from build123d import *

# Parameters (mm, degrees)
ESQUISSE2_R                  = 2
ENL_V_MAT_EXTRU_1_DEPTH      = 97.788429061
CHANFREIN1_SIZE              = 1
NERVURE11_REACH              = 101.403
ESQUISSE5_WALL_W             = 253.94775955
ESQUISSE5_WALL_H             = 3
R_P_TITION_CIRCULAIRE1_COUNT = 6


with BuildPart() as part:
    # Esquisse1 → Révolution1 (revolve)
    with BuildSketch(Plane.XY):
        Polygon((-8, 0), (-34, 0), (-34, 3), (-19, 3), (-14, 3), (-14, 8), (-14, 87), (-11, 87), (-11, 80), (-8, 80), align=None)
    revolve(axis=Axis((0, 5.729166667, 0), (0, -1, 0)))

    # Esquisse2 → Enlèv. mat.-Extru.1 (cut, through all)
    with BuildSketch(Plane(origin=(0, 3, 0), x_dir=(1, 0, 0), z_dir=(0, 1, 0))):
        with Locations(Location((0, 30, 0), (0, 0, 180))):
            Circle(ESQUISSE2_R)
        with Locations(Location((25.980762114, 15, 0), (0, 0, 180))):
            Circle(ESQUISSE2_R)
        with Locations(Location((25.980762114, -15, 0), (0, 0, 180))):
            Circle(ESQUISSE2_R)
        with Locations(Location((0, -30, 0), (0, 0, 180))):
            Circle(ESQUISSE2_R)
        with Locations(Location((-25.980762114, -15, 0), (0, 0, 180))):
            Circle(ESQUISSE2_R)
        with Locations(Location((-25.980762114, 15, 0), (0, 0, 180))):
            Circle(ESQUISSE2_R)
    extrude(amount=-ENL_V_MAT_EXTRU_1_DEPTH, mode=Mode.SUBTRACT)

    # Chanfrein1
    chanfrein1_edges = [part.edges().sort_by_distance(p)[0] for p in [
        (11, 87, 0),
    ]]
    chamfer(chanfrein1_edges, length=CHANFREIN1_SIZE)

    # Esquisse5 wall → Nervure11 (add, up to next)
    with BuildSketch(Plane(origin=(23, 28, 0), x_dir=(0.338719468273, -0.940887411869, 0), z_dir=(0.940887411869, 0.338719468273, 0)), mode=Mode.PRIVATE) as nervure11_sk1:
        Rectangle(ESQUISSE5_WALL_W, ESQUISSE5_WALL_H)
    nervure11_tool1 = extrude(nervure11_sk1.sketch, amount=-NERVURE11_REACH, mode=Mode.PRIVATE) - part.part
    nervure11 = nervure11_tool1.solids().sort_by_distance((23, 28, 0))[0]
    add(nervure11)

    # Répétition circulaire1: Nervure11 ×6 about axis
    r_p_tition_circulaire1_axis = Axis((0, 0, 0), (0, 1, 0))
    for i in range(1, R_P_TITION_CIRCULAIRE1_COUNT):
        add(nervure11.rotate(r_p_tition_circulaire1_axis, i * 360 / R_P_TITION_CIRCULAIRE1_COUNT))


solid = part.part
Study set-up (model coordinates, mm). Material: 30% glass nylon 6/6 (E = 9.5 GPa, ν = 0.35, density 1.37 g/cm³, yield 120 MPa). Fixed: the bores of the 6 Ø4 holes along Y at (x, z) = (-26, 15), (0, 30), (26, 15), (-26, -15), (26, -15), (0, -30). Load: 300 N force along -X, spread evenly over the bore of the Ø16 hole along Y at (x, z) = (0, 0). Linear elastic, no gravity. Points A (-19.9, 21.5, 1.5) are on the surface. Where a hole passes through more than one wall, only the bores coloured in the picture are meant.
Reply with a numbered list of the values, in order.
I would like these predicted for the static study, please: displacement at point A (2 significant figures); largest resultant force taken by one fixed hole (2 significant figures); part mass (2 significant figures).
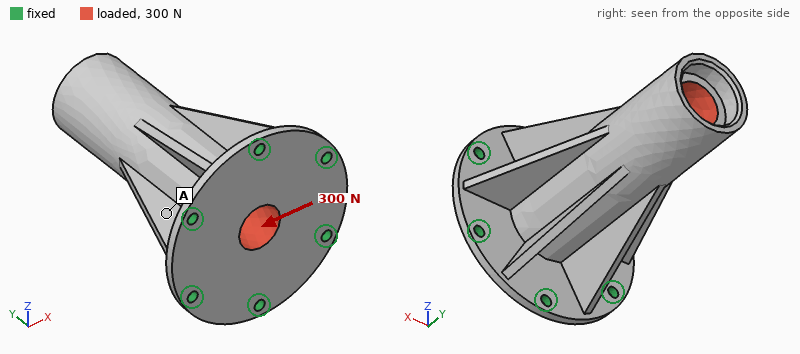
1. 0.059 mm
2. 130 N
3. 71 g
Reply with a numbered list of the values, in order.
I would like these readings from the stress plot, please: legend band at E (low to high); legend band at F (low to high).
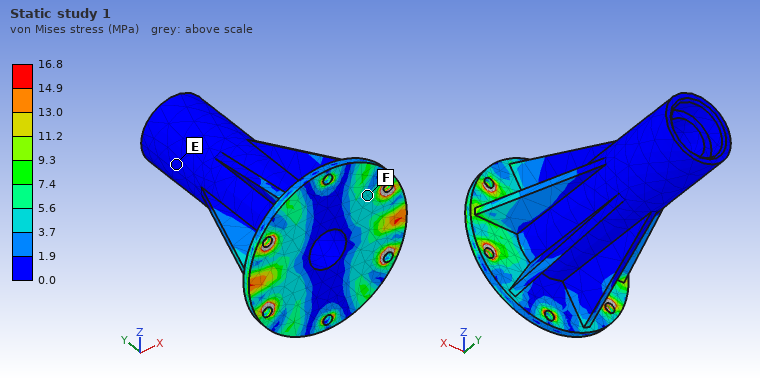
1. 0.0 to 1.9 MPa
2. 3.7 to 5.6 MPa
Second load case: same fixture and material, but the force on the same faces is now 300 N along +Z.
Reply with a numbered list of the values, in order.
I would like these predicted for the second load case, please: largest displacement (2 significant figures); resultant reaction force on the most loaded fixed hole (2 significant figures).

1. 0.20 mm
2. 150 N
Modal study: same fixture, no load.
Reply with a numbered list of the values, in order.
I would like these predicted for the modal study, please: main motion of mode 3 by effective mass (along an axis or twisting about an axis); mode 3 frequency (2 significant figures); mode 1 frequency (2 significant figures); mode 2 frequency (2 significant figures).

1. along Y
2. 2500 Hz
3. 1000 Hz
4. 1000 Hz
